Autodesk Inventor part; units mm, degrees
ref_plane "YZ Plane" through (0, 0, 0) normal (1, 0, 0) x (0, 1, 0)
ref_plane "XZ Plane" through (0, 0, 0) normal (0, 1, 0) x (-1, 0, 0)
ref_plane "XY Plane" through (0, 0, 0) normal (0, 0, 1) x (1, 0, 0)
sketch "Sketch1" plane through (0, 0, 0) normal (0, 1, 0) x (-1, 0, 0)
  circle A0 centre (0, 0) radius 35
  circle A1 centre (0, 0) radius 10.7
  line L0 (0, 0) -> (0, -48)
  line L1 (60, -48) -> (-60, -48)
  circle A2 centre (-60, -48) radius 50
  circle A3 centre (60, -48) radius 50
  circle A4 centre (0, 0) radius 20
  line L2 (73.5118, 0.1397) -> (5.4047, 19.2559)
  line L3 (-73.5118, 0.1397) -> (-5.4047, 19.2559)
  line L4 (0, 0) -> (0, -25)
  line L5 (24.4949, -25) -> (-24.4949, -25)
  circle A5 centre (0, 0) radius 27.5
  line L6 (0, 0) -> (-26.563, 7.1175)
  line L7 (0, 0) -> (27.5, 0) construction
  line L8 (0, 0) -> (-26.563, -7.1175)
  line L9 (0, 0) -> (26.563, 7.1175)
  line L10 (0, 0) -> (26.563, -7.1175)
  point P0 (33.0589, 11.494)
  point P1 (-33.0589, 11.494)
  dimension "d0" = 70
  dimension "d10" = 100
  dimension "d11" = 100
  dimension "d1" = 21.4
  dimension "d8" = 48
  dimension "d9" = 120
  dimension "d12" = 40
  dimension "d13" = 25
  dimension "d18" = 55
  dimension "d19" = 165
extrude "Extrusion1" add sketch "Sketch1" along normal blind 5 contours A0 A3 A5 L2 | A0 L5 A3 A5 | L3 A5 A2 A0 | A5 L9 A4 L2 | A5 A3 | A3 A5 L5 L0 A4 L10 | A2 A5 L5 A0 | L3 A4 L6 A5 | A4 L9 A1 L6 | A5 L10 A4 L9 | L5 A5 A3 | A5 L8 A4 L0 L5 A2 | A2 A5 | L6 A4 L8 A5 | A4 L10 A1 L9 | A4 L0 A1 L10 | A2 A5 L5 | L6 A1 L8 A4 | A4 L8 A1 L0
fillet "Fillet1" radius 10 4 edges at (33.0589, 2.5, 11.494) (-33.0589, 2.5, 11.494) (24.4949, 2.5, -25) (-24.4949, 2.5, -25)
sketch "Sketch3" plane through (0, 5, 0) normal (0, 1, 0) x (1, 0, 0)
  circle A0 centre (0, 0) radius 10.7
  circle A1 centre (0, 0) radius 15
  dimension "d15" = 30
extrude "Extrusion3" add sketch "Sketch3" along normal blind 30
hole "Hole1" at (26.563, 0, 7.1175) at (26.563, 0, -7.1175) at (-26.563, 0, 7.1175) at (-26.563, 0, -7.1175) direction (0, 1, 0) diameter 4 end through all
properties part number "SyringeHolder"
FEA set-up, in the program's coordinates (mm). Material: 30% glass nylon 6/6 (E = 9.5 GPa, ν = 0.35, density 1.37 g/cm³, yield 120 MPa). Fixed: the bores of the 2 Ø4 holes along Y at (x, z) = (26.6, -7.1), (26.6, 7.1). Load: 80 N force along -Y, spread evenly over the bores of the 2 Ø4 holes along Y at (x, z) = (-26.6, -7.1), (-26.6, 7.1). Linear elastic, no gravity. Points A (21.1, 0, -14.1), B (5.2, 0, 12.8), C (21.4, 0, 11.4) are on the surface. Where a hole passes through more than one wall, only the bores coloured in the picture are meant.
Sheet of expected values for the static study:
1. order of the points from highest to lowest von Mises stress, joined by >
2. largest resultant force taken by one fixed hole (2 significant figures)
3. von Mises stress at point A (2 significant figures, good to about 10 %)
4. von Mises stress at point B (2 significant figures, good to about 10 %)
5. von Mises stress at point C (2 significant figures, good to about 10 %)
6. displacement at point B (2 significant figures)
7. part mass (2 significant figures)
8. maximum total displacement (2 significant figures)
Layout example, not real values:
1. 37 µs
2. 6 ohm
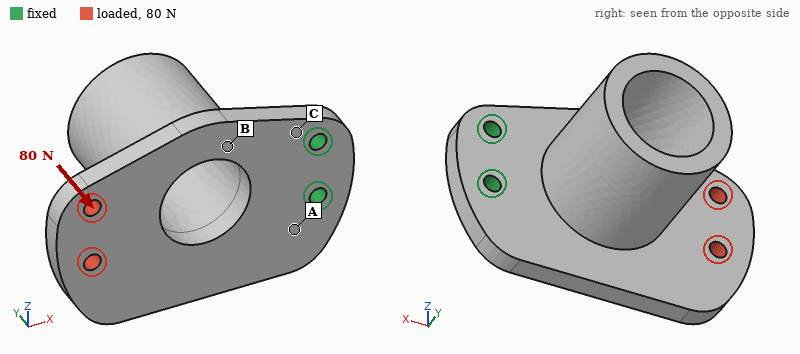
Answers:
1. C > A > B
2. 51 N
3. 18 MPa
4. 6.2 MPa
5. 26 MPa
6. 0.23 mm
7. 30 g
8. 0.99 mm
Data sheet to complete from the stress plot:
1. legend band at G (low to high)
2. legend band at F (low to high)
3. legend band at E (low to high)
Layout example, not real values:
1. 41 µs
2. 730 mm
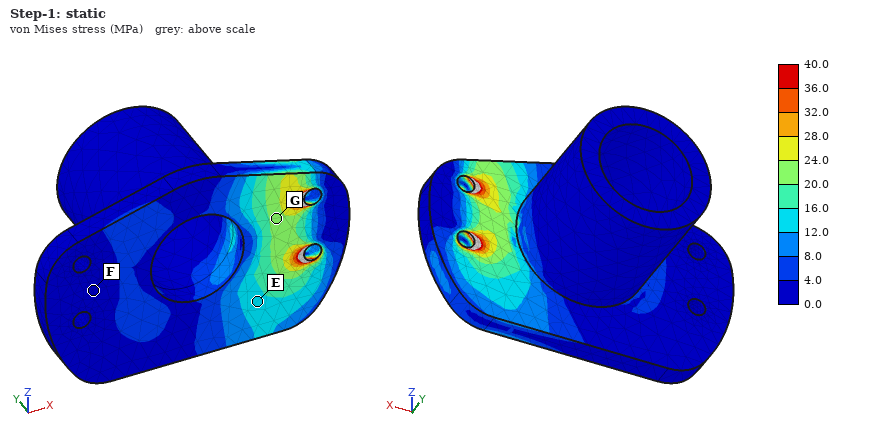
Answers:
1. 20.0 to 24.0 MPa
2. 0.0 to 4.0 MPa
3. 12.0 to 16.0 MPa
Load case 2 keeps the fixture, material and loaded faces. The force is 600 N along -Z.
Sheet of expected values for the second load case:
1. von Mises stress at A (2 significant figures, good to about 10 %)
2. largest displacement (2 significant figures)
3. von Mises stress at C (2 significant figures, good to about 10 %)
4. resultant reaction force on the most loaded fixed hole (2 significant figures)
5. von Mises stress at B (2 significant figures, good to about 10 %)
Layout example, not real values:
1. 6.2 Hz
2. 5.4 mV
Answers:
1. 14 MPa
2. 0.48 mm
3. 22 MPa
4. 1.8 kN
5. 21 MPa
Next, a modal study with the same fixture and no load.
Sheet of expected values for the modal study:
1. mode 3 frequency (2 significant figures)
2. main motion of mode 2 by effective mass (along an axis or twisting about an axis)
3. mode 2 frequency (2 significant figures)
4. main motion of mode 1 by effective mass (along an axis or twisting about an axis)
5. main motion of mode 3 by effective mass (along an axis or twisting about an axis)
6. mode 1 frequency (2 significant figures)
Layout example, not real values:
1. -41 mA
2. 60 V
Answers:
1. 2100 Hz
2. along Z
3. 1300 Hz
4. along Y
5. along Z
6. 490 Hz
